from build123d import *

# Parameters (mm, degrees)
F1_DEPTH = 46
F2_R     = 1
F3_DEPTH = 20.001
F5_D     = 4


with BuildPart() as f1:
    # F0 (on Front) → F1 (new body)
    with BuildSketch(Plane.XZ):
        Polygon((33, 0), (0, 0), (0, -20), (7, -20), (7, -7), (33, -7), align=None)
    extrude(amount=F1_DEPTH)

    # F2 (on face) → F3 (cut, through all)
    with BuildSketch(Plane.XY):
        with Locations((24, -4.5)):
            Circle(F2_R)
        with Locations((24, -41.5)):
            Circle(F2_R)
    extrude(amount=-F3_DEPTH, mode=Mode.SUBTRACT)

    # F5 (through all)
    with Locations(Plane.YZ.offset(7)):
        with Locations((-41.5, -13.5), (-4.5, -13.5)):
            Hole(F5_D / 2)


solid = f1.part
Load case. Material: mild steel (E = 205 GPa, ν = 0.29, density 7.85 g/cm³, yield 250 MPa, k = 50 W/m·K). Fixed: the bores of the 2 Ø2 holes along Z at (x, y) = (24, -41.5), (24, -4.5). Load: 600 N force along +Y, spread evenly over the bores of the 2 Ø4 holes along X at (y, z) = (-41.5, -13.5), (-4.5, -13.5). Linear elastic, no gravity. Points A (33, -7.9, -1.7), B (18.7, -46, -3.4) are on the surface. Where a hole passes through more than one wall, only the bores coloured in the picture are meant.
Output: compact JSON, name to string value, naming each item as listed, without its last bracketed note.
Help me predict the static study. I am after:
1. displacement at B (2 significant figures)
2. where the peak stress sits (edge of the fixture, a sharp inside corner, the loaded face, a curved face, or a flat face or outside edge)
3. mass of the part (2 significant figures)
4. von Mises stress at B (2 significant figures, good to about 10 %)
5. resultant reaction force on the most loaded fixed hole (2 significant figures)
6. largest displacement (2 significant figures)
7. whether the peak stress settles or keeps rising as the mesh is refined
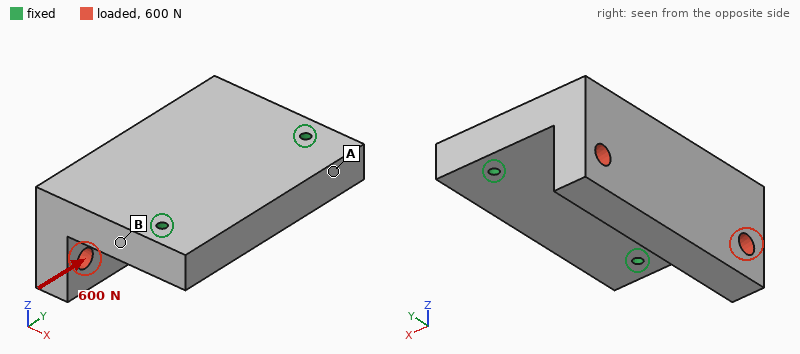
{"displacement at B": "0.71 µm", "where the peak stress sits": "edge of the fixture", "mass of the part": "110 g", "von Mises stress at B": "9.1 MPa", "resultant reaction force on the most loaded fixed hole": "470 N", "largest displacement": "4.7 µm", "whether the peak stress settles or keeps rising as the mesh is refined": "keeps rising"}
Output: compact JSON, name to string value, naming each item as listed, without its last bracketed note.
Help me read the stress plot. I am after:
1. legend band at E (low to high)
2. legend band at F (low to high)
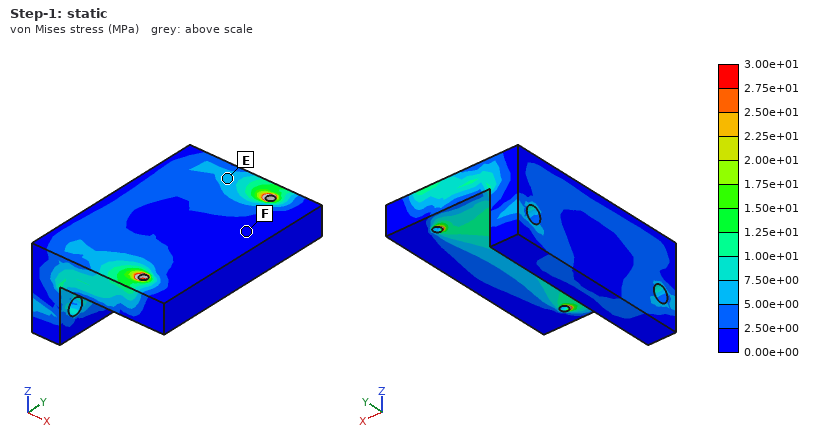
{"legend band at E": "5.00e+00 to 7.50e+00 MPa", "legend band at F": "0.00e+00 to 2.50e+00 MPa"}
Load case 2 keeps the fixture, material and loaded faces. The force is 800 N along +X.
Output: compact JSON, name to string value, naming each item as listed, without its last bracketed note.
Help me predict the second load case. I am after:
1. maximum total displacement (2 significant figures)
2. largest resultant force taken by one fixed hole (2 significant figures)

{"maximum total displacement": "21 µm", "largest resultant force taken by one fixed hole": "400 N"}
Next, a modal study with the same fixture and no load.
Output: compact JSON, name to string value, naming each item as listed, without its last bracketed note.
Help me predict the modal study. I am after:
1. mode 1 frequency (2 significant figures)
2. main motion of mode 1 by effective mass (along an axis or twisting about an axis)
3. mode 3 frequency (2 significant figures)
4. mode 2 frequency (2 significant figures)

{"mode 1 frequency": "4000 Hz", "main motion of mode 1 by effective mass": "along Z", "mode 3 frequency": "14 kHz", "mode 2 frequency": "8500 Hz"}
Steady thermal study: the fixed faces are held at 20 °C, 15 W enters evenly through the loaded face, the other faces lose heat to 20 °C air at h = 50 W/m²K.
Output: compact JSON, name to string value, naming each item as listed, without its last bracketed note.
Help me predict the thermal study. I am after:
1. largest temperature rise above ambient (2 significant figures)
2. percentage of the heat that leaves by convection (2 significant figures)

{"largest temperature rise above ambient": "33 K", "percentage of the heat that leaves by convection": "27 %"}
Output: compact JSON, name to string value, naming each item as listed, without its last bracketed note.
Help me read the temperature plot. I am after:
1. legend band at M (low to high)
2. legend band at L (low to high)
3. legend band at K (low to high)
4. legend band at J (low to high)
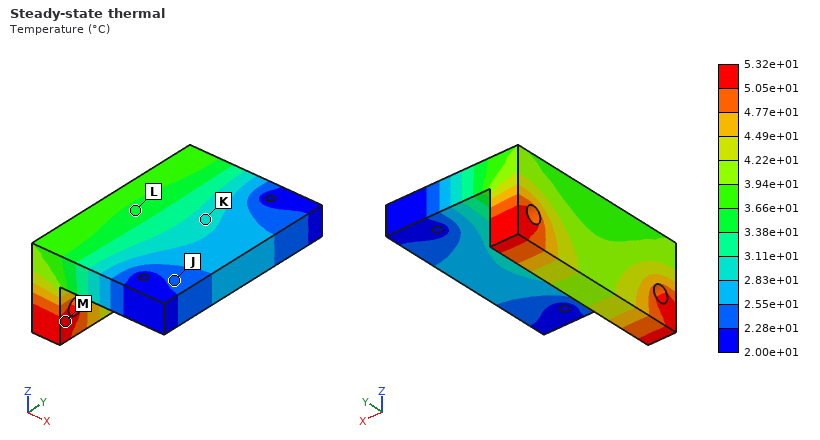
{"legend band at M": "5.05e+01 to 5.32e+01 °C", "legend band at L": "3.38e+01 to 3.66e+01 °C", "legend band at K": "2.83e+01 to 3.11e+01 °C", "legend band at J": "2.28e+01 to 2.55e+01 °C"}
